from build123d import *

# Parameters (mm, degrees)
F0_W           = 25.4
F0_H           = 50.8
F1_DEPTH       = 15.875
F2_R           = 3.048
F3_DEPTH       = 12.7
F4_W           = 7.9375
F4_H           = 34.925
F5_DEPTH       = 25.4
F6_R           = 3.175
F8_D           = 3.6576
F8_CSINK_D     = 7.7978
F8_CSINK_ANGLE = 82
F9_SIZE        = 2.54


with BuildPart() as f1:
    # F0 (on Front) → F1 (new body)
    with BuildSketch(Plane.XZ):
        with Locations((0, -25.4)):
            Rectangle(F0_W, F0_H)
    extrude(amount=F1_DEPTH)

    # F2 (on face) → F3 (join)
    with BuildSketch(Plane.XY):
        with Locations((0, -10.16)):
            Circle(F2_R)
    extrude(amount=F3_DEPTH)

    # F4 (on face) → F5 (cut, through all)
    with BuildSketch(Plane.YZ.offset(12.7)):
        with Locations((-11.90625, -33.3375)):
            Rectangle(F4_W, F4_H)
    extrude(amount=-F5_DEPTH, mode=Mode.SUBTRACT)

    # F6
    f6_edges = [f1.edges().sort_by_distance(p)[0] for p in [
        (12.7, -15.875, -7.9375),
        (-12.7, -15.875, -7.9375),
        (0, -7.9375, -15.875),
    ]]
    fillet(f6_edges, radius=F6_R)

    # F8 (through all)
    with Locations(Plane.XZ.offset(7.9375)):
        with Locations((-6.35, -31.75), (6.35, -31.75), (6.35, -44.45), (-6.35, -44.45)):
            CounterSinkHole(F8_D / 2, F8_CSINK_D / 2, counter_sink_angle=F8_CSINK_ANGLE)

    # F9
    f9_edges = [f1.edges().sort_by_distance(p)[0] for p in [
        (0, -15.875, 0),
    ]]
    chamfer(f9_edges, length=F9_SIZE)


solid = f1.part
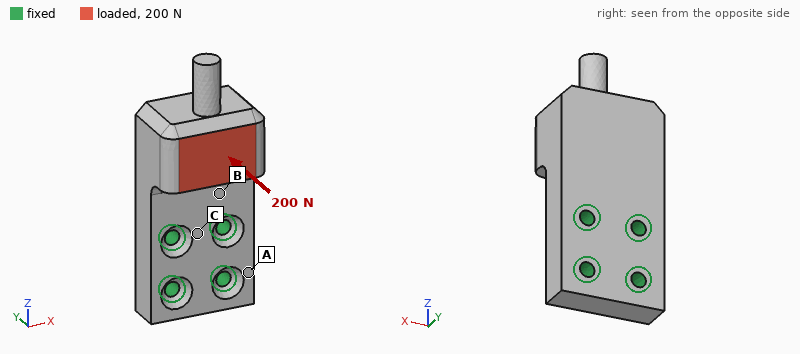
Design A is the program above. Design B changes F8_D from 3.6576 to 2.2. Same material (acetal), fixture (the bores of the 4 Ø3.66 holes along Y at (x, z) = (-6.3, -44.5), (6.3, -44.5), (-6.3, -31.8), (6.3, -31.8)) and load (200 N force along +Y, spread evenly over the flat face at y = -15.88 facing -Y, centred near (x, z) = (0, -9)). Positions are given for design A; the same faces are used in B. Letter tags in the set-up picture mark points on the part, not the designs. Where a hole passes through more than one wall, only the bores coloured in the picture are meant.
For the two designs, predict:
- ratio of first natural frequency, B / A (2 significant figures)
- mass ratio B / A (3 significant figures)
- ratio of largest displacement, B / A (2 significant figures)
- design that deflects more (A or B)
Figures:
0.90
1.01
1.2
B
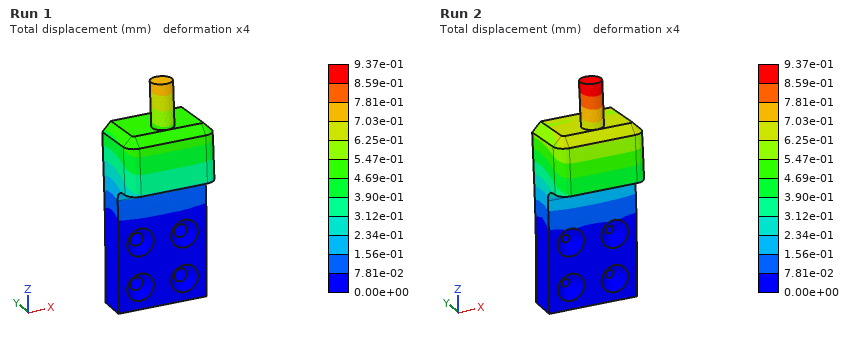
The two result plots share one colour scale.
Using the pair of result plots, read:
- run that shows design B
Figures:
Run 2
